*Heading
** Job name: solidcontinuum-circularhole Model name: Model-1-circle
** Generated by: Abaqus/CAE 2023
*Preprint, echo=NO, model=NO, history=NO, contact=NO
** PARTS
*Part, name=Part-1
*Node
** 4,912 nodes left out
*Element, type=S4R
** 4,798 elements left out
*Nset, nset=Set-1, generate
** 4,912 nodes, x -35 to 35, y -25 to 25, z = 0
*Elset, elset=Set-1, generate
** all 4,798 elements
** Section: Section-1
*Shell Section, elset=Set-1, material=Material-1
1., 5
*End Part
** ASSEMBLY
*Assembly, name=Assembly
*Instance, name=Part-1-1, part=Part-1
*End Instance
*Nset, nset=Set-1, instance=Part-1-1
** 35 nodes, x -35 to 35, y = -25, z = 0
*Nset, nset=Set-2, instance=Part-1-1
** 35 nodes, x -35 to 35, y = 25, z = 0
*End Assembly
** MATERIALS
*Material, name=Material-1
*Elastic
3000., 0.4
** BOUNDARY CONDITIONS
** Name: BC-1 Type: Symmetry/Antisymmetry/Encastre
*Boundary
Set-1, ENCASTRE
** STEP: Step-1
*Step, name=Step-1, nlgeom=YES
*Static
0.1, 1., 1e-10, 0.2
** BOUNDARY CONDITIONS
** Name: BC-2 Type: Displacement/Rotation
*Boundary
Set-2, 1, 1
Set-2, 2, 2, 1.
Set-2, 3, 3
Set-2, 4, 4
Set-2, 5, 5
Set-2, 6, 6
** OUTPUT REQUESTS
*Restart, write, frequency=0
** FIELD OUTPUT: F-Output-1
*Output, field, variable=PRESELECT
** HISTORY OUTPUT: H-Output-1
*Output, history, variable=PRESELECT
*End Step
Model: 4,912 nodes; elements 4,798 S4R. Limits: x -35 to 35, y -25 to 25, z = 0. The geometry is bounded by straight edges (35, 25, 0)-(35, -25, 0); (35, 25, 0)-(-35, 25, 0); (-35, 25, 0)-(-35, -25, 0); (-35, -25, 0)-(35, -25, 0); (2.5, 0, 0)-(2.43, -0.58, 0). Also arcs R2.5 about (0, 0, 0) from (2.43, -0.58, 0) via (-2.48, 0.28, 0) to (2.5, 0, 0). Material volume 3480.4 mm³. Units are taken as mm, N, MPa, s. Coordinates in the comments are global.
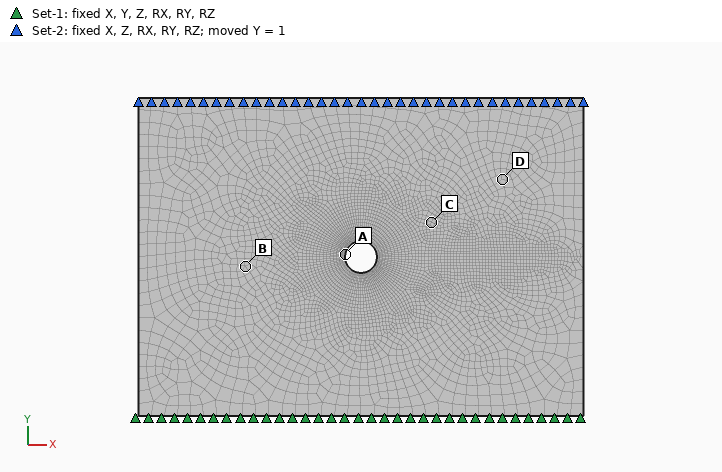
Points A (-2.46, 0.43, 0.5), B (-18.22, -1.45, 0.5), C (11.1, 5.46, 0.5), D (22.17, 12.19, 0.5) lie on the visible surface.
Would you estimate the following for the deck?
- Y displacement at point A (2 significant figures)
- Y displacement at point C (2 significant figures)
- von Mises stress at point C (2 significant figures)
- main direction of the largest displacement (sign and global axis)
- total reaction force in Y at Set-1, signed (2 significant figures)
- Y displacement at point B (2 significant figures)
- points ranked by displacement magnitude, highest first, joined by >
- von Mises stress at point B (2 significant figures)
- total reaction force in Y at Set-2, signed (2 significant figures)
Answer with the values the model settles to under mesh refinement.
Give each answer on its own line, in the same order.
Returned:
0.53 mm
0.62 mm
69 MPa
+Y
-4500 N
0.47 mm
D > C > A > B
67 MPa
4500 N
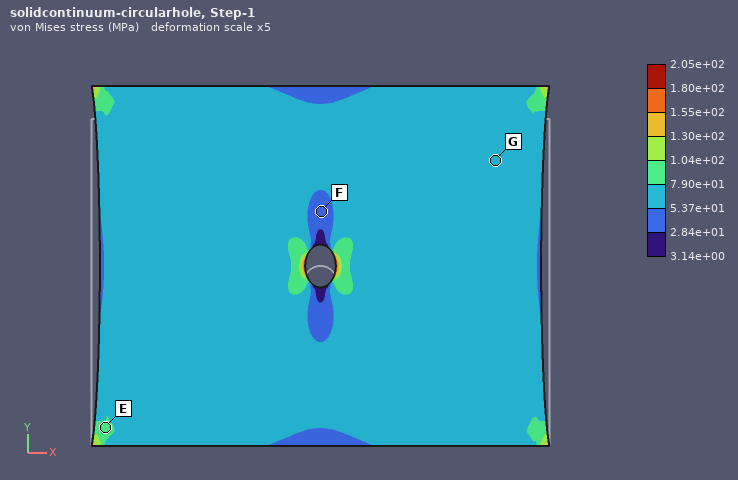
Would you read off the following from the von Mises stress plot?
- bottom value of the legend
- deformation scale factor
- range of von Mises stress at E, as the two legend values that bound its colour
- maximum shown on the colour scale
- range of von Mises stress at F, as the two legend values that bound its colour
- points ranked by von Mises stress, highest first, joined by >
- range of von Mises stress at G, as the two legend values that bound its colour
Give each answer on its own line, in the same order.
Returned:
3.14e+00 MPa
5
7.90e+01 to 1.04e+02 MPa
2.05e+02 MPa
2.84e+01 to 5.37e+01 MPa
E > G > F
5.37e+01 to 7.90e+01 MPa
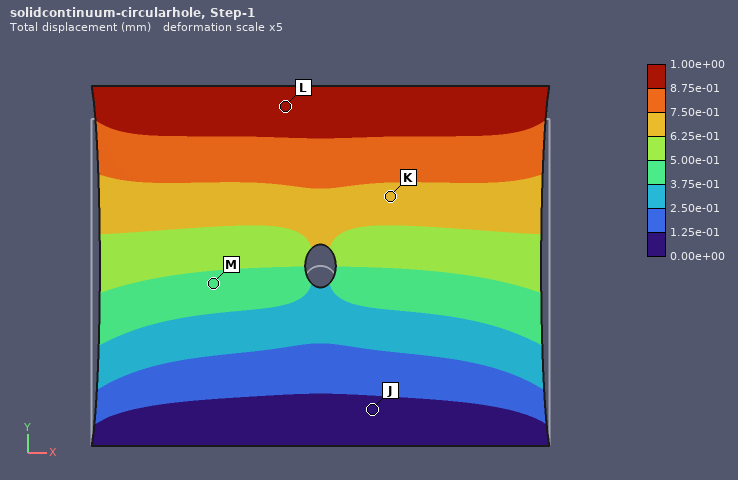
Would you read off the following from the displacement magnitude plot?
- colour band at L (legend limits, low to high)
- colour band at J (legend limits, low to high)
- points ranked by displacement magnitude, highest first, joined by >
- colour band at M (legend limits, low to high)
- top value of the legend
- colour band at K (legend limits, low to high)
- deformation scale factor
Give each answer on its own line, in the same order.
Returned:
8.75e-01 to 1.00e+00 mm
0.00e+00 to 1.25e-01 mm
L > K > M > J
3.75e-01 to 5.00e-01 mm
1.00e+00 mm
6.25e-01 to 7.50e-01 mm
5
